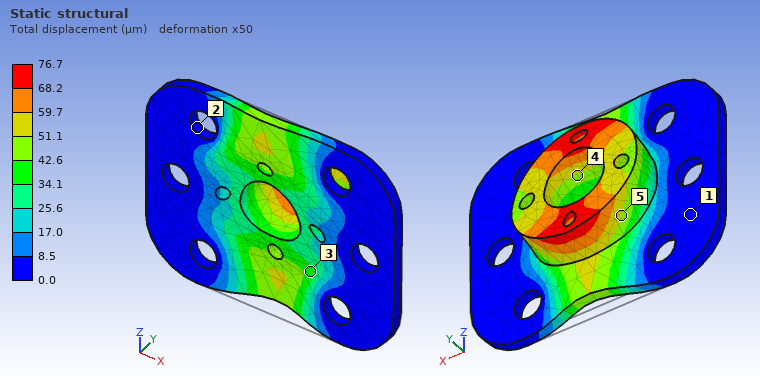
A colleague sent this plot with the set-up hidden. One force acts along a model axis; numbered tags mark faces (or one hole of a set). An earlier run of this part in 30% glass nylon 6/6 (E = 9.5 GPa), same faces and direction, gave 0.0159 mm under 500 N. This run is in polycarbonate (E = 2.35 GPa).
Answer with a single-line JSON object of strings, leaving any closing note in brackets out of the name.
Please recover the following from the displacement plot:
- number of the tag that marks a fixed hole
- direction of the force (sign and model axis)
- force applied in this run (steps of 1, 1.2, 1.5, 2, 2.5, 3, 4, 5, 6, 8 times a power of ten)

{"number of the tag that marks a fixed hole": "2", "direction of the force": "+Z", "force applied in this run": "600 N"}
